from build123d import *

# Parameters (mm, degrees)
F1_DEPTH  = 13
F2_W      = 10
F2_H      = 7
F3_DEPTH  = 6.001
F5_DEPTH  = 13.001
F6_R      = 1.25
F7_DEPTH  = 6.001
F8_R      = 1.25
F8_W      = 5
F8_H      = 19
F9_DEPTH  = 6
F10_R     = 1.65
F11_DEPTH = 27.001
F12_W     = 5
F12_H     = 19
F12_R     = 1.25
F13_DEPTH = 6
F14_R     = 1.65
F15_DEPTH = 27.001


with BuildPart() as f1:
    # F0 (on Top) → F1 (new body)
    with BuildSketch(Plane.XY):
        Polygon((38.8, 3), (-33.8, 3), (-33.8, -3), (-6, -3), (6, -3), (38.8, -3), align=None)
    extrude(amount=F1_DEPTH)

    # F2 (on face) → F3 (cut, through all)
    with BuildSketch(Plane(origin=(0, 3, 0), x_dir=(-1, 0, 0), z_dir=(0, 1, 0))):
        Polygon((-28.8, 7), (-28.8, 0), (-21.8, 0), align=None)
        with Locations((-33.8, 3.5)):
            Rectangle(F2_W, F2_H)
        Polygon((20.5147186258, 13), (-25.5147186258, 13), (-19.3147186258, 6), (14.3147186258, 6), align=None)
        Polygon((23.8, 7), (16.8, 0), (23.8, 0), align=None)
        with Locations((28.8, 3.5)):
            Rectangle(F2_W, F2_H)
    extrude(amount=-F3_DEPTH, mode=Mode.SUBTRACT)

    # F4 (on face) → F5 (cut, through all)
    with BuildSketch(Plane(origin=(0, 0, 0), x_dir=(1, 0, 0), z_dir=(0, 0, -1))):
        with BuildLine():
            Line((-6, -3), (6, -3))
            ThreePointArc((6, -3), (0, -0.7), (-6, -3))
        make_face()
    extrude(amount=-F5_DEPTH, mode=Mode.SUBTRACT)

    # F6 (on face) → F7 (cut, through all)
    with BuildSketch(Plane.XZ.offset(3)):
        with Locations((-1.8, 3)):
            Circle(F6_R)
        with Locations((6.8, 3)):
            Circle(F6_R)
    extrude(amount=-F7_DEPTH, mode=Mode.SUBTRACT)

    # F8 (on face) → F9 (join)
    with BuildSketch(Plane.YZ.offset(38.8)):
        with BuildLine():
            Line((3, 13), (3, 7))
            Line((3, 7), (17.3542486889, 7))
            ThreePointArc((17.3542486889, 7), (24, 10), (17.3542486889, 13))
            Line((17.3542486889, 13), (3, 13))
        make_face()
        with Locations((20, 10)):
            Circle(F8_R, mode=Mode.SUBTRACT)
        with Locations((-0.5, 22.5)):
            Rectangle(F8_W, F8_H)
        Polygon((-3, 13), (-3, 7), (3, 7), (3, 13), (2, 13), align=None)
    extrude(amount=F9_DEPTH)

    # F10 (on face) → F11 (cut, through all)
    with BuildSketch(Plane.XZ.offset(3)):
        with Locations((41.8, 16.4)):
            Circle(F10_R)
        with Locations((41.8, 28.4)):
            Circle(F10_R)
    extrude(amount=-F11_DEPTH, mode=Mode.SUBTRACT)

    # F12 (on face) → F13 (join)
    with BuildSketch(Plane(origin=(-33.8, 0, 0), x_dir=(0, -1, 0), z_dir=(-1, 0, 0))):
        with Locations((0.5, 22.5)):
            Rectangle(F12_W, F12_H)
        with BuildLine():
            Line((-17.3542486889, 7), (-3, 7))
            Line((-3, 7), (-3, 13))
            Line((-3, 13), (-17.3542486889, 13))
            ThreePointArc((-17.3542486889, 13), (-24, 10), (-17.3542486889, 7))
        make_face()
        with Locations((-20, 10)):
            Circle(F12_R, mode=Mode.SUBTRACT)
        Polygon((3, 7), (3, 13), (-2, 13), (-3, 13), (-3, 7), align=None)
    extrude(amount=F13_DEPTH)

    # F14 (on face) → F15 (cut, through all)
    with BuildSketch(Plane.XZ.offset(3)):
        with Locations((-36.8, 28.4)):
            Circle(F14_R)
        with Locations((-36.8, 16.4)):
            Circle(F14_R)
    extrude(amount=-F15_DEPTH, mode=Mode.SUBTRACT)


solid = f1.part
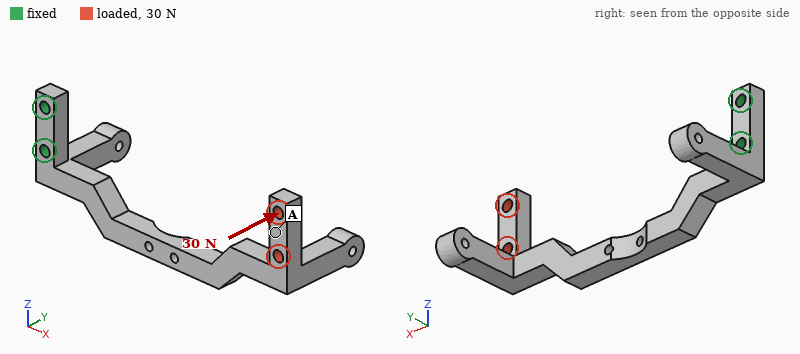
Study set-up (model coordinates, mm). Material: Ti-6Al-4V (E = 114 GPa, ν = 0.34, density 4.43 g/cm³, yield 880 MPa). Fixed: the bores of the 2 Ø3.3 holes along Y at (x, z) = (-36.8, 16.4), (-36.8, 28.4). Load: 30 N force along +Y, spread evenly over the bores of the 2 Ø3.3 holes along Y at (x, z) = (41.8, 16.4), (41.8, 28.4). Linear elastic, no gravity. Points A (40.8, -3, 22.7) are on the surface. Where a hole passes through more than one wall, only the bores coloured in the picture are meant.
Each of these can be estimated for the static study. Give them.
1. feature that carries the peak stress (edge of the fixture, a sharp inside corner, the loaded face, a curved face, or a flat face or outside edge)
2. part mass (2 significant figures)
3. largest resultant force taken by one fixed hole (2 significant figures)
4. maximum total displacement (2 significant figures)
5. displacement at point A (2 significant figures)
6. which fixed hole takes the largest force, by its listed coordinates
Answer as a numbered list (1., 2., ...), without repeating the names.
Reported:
1. a curved face
2. 25 g
3. 29 N
4. 0.91 mm
5. 0.79 mm
6. (-36.8, 16.4)
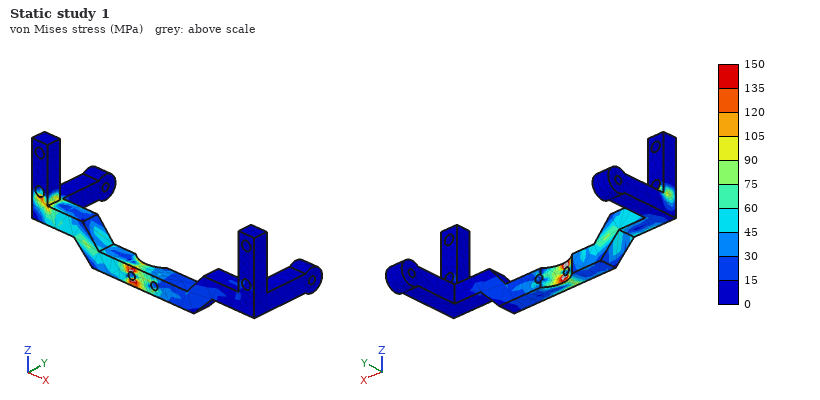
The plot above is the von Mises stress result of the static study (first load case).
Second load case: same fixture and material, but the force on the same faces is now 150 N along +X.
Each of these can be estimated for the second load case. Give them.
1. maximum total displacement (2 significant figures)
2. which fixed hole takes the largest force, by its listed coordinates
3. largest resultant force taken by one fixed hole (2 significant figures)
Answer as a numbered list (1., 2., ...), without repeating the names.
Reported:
1. 0.93 mm
2. (-36.8, 16.4)
3. 140 N
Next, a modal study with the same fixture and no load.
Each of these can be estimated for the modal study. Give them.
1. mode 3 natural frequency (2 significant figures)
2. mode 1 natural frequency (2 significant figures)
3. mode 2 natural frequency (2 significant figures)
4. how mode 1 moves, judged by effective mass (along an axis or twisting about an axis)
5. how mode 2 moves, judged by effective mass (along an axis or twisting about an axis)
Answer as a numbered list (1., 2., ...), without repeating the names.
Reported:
1. 1400 Hz
2. 340 Hz
3. 390 Hz
4. along Y
5. along Z
